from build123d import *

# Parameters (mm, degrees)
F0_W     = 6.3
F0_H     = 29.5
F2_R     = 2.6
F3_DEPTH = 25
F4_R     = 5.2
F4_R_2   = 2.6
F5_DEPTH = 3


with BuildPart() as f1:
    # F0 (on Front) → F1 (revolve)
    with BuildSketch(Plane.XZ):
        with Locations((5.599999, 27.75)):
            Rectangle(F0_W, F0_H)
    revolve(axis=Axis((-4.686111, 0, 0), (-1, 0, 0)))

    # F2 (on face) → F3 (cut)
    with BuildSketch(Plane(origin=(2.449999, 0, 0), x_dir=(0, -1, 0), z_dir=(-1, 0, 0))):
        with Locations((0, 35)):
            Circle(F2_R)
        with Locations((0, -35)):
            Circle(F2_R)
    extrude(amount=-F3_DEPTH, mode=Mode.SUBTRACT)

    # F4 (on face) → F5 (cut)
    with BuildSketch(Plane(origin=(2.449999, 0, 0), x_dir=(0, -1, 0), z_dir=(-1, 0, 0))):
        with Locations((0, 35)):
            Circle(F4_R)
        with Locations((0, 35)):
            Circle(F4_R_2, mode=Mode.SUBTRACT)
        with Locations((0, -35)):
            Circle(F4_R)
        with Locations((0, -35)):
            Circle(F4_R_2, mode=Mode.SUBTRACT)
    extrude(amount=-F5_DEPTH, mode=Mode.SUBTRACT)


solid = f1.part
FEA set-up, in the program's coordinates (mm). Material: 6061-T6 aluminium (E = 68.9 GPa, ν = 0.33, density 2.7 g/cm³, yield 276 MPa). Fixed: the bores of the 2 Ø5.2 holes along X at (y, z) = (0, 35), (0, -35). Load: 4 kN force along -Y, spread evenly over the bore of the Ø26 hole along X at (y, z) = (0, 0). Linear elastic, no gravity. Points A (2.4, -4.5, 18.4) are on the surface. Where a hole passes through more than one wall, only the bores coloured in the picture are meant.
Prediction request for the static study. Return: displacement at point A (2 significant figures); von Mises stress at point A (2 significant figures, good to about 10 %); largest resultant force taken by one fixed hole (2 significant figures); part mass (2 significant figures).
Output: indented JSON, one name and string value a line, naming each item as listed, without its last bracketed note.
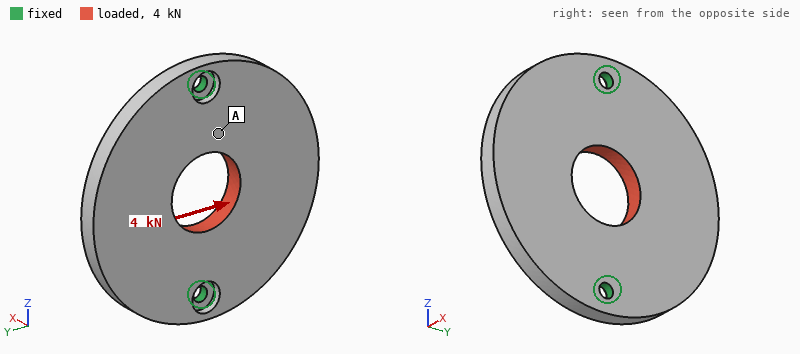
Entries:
{
  "displacement at point A": "13 µm",
  "von Mises stress at point A": "11 MPa",
  "largest resultant force taken by one fixed hole": "2.0 kN",
  "part mass": "86 g"
}
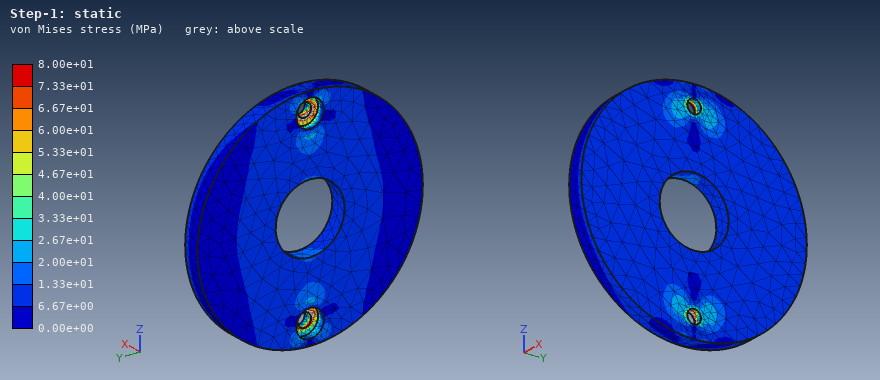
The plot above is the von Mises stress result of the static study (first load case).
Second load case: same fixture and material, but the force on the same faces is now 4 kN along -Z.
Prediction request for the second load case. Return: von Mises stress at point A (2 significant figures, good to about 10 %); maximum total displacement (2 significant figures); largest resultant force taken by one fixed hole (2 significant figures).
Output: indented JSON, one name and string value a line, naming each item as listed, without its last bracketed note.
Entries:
{
  "von Mises stress at point A": "10 MPa",
  "maximum total displacement": "8.9 µm",
  "largest resultant force taken by one fixed hole": "2.0 kN"
}
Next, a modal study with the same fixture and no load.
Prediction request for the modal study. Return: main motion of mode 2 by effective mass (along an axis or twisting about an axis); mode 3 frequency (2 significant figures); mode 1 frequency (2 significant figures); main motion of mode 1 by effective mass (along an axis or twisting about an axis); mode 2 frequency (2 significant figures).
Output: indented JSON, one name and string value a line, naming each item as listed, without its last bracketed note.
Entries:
{
  "main motion of mode 2 by effective mass": "along X",
  "mode 3 frequency": "5300 Hz",
  "mode 1 frequency": "1600 Hz",
  "main motion of mode 1 by effective mass": "twisting about Z",
  "mode 2 frequency": "2500 Hz"
}
